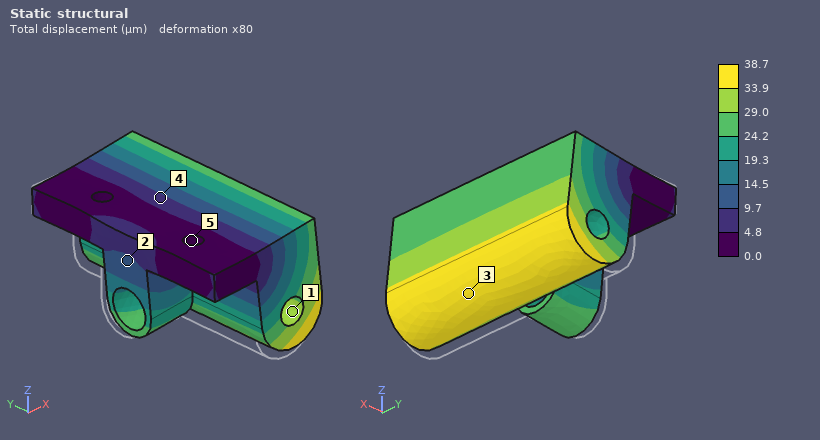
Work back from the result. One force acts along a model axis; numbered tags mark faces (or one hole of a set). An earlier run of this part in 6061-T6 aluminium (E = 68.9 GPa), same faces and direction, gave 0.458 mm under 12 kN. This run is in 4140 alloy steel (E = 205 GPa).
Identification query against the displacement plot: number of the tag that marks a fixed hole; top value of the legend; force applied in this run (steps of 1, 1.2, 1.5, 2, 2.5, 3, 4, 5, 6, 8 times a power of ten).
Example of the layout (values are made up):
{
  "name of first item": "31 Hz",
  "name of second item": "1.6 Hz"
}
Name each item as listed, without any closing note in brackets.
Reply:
{
  "number of the tag that marks a fixed hole": "5",
  "top value of the legend": "38.7 µm",
  "force applied in this run": "3 kN"
}
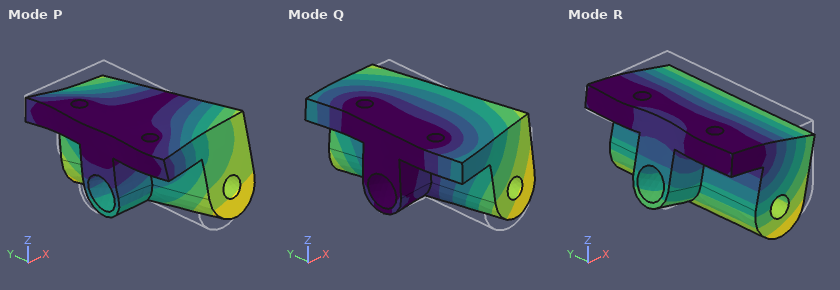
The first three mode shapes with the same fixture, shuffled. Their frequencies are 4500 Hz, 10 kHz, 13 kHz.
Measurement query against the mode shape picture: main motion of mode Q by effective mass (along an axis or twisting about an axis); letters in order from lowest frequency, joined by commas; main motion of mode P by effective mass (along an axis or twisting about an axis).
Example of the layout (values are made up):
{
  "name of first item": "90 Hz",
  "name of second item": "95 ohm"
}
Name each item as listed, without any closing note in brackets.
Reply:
{
  "main motion of mode Q by effective mass": "along Y",
  "letters in order from lowest frequency, joined by commas": "R, P, Q",
  "main motion of mode P by effective mass": "along Y"
}
